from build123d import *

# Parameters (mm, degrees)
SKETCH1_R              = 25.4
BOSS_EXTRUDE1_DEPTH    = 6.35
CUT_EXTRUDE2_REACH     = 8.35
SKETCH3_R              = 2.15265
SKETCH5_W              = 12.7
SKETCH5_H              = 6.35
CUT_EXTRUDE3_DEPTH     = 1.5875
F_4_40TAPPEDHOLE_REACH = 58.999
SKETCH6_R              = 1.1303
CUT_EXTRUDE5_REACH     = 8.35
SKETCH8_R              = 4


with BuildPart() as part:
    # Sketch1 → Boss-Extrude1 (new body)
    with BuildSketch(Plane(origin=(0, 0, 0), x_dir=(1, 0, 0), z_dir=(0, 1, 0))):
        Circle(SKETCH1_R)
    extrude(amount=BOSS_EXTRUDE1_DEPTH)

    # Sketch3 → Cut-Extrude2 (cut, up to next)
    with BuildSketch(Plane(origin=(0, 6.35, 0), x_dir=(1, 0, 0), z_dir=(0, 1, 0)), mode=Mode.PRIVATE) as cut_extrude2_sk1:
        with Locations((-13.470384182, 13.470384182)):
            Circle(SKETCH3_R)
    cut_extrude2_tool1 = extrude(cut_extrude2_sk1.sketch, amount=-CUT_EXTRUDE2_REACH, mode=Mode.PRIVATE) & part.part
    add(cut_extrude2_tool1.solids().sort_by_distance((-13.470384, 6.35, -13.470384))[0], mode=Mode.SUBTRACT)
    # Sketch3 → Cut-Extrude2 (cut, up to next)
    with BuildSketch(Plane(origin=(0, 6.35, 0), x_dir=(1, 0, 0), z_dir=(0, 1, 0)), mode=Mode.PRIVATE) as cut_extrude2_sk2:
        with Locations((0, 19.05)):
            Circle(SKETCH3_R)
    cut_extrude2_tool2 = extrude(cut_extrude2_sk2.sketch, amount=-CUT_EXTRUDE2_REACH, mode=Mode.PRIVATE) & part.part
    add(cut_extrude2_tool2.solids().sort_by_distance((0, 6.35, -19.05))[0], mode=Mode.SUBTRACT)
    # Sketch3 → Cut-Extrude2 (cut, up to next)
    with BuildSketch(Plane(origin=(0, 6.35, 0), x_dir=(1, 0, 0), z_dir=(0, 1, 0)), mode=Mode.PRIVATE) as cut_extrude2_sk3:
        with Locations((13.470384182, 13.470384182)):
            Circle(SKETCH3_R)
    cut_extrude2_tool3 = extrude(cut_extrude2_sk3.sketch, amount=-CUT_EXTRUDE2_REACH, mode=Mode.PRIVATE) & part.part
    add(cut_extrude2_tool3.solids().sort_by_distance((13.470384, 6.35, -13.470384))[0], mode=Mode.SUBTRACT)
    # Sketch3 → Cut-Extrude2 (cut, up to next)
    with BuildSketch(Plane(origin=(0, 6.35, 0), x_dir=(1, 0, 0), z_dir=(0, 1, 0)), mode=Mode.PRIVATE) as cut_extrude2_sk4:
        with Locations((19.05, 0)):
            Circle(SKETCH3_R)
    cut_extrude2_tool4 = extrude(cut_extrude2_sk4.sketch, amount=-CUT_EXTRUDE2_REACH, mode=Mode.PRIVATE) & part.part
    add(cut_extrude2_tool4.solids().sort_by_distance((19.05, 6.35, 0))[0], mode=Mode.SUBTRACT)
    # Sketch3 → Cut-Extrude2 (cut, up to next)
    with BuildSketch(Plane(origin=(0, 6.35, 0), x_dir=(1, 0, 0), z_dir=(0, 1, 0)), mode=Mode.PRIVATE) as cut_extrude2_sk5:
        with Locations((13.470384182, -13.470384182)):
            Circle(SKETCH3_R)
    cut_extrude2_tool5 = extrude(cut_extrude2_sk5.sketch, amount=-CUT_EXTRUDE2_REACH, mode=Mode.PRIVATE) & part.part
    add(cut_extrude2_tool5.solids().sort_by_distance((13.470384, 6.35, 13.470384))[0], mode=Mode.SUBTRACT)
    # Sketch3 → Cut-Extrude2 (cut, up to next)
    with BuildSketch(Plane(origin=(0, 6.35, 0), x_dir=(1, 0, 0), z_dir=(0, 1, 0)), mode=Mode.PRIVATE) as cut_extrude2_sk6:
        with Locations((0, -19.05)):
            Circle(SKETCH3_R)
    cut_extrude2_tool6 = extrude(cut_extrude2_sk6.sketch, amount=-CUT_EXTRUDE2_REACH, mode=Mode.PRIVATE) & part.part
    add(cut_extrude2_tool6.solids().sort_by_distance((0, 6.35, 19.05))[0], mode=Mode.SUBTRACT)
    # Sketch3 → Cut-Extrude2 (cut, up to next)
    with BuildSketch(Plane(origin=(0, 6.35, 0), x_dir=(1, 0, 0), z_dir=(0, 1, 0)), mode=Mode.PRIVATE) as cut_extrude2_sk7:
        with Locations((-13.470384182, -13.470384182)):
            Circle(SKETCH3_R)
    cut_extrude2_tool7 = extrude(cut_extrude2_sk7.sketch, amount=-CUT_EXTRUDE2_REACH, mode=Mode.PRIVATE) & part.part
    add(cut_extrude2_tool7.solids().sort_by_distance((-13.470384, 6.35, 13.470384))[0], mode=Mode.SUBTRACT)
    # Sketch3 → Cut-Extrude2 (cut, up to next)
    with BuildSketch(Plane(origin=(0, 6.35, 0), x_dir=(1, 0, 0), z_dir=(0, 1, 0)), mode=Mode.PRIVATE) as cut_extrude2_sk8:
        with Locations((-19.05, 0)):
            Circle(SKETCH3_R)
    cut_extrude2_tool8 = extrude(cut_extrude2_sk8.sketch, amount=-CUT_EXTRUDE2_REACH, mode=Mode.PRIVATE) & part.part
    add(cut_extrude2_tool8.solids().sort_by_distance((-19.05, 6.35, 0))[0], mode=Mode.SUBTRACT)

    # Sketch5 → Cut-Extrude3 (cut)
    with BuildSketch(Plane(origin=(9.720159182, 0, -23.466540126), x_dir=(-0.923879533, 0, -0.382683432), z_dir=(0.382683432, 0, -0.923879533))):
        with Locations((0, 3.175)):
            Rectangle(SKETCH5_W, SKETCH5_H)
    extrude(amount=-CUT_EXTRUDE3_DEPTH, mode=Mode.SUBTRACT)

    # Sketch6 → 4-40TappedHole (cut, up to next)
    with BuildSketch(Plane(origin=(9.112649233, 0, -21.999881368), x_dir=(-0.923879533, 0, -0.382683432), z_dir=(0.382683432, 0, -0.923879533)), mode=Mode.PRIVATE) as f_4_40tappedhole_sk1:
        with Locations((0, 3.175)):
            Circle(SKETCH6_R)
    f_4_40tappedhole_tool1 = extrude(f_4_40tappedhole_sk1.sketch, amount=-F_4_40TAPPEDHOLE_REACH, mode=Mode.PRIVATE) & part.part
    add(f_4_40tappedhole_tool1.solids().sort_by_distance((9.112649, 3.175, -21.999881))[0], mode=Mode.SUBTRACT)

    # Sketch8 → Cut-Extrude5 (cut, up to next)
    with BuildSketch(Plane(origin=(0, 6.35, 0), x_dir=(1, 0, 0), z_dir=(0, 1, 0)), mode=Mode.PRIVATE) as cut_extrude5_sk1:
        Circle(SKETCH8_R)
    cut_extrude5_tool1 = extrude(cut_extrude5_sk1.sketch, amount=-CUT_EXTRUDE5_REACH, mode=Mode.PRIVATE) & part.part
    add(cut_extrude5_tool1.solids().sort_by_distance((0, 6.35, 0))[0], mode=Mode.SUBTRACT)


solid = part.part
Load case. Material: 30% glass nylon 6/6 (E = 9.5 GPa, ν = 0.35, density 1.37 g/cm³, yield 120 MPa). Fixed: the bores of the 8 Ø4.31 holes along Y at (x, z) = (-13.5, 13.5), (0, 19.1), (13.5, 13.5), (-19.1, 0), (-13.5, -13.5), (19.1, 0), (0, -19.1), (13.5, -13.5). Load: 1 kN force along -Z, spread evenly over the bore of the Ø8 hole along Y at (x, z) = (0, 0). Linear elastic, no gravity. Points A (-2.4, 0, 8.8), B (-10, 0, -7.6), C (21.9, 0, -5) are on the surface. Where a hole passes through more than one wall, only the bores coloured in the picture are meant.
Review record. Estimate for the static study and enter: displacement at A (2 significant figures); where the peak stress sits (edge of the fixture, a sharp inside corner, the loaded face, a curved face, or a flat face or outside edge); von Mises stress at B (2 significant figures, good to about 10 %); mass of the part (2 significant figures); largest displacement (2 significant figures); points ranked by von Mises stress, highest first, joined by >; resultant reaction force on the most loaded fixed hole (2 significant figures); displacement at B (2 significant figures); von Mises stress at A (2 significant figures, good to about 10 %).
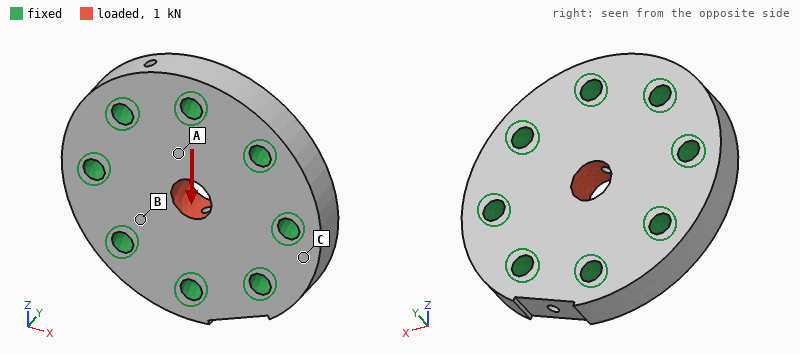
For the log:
3.6 µm
the loaded face
2.6 MPa
16 g
7.2 µm
A > B > C
220 N
1.4 µm
4.5 MPa
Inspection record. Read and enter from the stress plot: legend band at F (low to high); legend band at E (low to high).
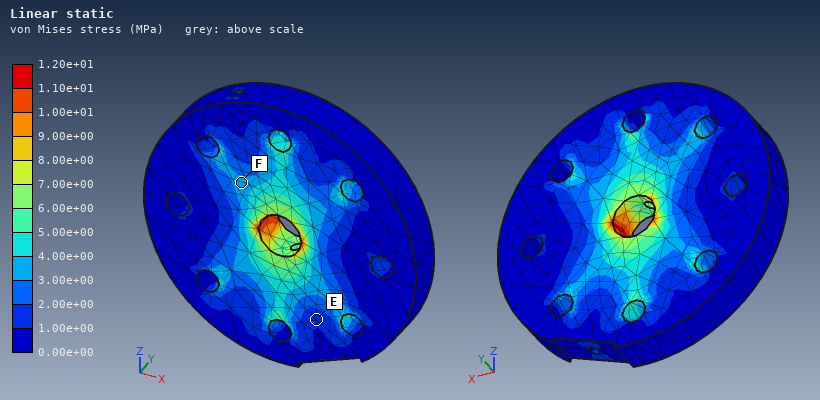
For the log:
3.00e+00 to 4.00e+00 MPa
1.00e+00 to 2.00e+00 MPa
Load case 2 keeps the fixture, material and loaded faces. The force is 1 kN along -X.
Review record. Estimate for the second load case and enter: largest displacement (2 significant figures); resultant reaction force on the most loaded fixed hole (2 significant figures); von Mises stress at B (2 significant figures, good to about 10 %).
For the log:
7.4 µm
230 N
2.8 MPa
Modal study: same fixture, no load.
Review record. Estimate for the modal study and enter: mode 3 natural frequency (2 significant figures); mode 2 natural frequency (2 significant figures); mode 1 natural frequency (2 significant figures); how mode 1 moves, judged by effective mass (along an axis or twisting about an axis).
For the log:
31 kHz
30 kHz
19 kHz
along Y
